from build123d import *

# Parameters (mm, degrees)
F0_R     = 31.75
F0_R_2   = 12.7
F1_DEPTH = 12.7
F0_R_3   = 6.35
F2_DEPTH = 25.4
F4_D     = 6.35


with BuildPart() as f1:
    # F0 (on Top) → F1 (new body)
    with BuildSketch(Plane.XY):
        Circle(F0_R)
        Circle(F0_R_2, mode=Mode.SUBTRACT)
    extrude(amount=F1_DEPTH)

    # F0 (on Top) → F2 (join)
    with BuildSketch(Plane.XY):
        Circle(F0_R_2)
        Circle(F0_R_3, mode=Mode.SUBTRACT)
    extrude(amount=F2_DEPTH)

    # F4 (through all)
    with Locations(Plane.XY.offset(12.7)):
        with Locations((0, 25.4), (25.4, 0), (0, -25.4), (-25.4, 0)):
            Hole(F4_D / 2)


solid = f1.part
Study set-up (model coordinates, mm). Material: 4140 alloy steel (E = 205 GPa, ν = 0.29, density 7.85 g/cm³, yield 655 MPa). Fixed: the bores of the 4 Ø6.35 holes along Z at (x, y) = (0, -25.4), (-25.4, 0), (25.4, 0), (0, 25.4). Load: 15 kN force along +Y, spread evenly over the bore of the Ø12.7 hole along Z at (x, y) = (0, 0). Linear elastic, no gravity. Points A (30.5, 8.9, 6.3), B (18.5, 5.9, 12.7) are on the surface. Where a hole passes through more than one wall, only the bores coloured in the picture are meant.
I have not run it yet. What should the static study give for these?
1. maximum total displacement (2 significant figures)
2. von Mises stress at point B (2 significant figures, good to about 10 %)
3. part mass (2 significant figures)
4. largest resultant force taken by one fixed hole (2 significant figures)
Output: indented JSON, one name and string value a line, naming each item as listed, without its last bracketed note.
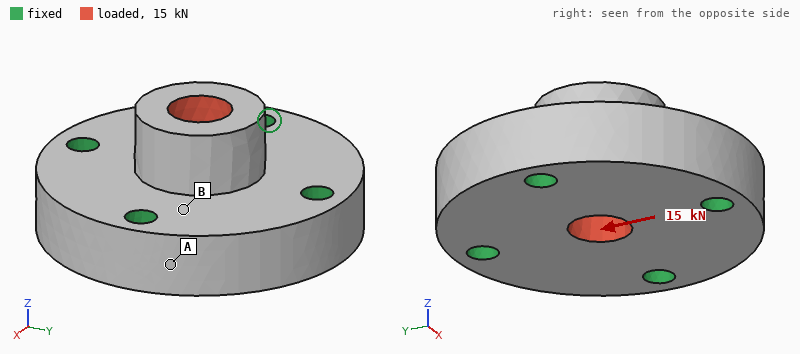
{
  "maximum total displacement": "8.3 µm",
  "von Mises stress at point B": "13 MPa",
  "part mass": "330 g",
  "largest resultant force taken by one fixed hole": "5.3 kN"
}
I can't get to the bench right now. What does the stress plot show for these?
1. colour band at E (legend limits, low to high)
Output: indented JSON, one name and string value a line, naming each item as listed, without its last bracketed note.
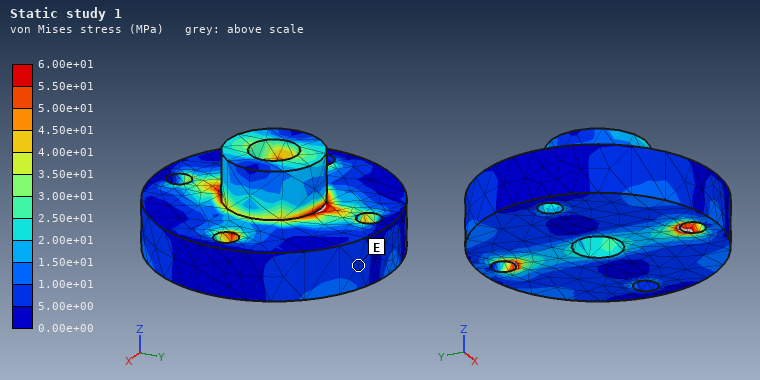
{
  "colour band at E": "5.00e+00 to 1.00e+01 MPa"
}
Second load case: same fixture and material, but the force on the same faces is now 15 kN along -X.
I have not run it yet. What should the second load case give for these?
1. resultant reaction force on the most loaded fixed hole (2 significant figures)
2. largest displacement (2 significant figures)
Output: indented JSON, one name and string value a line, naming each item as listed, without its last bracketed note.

{
  "resultant reaction force on the most loaded fixed hole": "5.3 kN",
  "largest displacement": "8.3 µm"
}
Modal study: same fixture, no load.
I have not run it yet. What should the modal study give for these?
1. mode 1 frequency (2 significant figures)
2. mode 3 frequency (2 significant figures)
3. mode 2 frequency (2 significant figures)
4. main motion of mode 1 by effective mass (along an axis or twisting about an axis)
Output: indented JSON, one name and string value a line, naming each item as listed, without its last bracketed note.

{
  "mode 1 frequency": "25 kHz",
  "mode 3 frequency": "26 kHz",
  "mode 2 frequency": "26 kHz",
  "main motion of mode 1 by effective mass": "along Z"
}
